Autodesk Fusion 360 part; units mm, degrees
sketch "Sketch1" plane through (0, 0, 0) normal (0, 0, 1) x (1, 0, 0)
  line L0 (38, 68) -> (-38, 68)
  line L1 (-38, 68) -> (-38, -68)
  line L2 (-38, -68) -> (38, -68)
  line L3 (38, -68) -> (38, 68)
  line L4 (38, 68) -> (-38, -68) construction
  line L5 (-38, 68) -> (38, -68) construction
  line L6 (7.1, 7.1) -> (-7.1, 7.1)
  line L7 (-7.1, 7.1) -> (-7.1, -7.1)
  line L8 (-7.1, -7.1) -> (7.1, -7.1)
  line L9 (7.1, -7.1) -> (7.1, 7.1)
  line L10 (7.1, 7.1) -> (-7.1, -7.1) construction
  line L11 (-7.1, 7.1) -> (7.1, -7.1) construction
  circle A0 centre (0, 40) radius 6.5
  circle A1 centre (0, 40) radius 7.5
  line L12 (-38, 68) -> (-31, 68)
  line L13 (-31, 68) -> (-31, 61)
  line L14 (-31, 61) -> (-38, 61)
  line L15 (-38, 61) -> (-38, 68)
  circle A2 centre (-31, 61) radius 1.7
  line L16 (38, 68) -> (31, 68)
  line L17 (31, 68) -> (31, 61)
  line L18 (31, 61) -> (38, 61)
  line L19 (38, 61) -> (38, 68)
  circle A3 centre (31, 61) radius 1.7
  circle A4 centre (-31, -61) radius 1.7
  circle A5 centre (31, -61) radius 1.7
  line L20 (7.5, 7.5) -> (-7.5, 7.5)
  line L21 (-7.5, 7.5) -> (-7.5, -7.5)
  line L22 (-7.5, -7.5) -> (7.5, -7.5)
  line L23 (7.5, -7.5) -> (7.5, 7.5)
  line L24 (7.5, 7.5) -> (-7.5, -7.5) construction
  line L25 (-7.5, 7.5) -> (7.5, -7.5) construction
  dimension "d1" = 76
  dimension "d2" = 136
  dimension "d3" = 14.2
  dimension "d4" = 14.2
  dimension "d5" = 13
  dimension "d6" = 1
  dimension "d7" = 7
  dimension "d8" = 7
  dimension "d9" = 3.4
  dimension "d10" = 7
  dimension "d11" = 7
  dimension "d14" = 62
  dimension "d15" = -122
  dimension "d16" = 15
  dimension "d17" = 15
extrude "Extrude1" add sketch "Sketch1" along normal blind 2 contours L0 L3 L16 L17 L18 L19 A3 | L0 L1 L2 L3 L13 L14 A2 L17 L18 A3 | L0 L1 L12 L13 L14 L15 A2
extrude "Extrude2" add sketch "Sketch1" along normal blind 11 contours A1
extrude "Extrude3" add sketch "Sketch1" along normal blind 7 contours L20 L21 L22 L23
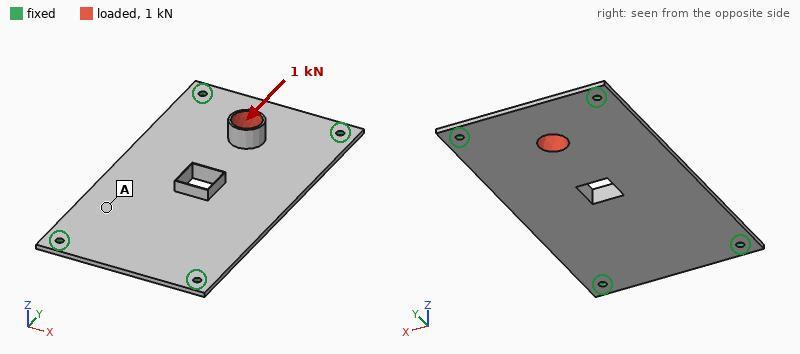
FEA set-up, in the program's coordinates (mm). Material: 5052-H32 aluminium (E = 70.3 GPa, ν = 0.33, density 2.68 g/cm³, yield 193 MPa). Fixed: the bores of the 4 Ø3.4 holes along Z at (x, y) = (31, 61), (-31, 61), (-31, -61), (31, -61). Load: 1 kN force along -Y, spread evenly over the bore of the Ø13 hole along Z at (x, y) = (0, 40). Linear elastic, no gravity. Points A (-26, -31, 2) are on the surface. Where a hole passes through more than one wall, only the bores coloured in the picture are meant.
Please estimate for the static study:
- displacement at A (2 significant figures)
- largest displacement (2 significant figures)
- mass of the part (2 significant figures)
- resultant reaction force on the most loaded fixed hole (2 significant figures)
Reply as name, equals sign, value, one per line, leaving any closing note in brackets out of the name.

displacement at A = 0.13 mm
largest displacement = 0.33 mm
mass of the part = 55 g
resultant reaction force on the most loaded fixed hole = 370 N
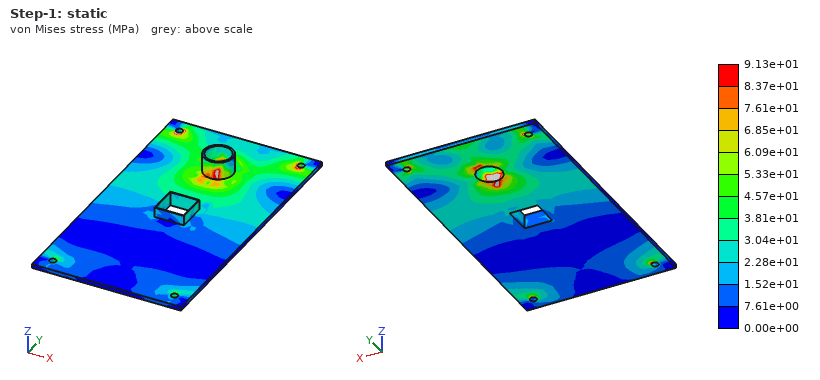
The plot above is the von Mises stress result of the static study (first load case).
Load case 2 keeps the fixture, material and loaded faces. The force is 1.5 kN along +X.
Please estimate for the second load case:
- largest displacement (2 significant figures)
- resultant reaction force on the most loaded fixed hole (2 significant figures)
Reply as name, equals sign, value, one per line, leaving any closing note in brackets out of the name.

largest displacement = 0.21 mm
resultant reaction force on the most loaded fixed hole = 690 N
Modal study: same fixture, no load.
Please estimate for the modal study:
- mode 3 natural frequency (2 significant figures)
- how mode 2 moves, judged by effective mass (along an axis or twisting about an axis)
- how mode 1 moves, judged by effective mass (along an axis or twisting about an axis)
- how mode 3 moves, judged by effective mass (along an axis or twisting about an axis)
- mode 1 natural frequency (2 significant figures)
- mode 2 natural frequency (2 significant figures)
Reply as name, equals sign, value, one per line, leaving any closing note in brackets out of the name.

mode 3 natural frequency = 1700 Hz
how mode 2 moves, judged by effective mass = twisting about Y
how mode 1 moves, judged by effective mass = along Z
how mode 3 moves, judged by effective mass = twisting about X
mode 1 natural frequency = 630 Hz
mode 2 natural frequency = 1000 Hz
